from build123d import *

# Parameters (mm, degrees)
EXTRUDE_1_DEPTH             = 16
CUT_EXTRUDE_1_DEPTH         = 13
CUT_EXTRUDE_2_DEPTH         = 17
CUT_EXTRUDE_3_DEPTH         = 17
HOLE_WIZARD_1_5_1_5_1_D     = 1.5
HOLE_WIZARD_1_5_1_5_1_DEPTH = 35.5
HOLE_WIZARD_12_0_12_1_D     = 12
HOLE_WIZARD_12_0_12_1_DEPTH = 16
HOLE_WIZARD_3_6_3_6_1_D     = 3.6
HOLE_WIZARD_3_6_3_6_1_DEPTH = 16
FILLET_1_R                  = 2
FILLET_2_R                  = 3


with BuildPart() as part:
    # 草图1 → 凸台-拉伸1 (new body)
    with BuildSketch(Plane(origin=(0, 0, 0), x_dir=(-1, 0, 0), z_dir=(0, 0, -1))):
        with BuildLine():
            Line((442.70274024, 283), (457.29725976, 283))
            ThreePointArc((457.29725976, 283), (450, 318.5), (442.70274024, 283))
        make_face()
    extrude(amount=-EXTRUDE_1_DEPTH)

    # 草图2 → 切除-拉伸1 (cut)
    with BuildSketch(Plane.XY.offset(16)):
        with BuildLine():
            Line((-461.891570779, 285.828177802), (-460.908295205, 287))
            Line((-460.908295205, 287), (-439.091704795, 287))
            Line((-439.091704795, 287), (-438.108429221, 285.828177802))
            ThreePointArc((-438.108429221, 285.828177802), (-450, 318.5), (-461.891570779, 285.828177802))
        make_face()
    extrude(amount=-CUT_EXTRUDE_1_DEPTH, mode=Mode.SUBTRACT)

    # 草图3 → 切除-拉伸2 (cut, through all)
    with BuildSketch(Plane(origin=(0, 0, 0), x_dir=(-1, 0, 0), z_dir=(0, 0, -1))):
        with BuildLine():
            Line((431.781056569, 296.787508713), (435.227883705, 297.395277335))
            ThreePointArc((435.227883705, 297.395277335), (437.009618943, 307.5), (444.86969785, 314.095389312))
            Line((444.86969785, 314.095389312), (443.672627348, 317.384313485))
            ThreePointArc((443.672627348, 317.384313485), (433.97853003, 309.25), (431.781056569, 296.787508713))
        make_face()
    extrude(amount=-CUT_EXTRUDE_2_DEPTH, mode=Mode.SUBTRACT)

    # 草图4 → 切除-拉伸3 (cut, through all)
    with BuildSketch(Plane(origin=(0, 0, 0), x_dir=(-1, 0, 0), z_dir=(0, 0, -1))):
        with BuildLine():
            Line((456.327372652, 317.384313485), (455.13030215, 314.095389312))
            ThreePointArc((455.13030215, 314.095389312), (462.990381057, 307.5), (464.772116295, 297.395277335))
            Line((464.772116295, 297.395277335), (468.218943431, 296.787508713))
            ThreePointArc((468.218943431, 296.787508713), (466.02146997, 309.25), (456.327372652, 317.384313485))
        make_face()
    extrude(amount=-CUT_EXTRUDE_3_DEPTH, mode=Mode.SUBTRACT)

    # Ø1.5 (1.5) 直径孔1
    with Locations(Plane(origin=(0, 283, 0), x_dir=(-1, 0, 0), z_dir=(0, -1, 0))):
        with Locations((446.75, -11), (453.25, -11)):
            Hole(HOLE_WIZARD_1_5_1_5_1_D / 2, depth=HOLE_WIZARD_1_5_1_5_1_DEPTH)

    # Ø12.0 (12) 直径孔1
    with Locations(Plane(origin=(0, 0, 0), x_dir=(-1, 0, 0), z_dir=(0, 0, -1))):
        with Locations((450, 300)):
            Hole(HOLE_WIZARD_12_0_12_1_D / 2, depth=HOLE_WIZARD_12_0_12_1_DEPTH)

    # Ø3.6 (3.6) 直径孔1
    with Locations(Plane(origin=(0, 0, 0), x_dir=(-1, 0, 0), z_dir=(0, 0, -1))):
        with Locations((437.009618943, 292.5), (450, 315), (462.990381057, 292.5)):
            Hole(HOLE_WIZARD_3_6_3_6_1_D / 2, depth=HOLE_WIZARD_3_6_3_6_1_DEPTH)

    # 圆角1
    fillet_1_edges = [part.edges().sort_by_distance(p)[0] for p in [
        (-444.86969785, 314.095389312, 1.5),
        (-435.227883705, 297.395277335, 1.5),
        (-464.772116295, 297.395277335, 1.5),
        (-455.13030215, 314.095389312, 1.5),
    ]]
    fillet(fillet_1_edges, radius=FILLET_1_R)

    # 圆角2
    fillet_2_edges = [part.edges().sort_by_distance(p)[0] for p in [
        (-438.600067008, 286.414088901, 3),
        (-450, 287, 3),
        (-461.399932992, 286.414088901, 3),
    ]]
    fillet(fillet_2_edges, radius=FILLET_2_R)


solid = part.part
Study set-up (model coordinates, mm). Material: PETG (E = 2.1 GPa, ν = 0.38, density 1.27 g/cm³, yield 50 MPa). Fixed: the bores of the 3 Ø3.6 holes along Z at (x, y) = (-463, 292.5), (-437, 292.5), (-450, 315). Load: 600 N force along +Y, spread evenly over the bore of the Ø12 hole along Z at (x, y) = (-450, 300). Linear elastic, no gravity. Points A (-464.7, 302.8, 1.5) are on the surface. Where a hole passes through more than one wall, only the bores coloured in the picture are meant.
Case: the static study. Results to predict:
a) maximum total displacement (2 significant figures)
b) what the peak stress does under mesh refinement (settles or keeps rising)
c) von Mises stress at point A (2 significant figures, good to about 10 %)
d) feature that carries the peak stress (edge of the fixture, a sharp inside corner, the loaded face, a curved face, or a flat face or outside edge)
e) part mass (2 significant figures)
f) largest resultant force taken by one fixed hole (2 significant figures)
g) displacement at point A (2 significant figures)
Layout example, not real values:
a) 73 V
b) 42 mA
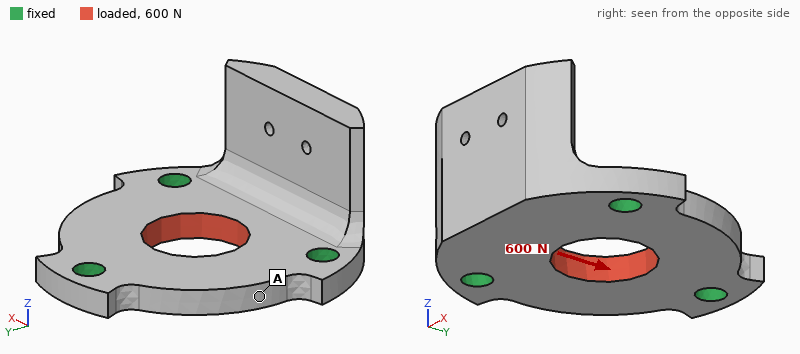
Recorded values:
a) 68 µm
b) keeps rising
c) 3.9 MPa
d) edge of the fixture
e) 4.3 g
f) 200 N
g) 24 µm
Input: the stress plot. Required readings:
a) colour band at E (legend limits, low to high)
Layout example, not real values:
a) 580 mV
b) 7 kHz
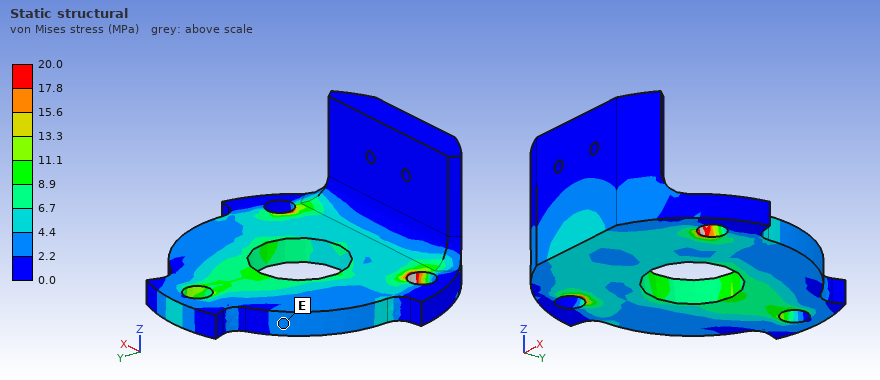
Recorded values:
a) 2.2 to 4.4 MPa
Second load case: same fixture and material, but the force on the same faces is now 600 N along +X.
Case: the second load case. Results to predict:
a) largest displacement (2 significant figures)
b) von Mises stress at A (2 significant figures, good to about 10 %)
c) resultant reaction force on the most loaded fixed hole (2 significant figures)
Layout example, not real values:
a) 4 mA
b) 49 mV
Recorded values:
a) 78 µm
b) 5.6 MPa
c) 200 N
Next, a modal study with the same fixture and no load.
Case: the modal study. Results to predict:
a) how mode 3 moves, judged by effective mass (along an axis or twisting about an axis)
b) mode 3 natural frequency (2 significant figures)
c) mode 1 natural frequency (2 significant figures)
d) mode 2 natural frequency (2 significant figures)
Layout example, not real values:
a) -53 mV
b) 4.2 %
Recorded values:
a) along Z
b) 5300 Hz
c) 1800 Hz
d) 4600 Hz
